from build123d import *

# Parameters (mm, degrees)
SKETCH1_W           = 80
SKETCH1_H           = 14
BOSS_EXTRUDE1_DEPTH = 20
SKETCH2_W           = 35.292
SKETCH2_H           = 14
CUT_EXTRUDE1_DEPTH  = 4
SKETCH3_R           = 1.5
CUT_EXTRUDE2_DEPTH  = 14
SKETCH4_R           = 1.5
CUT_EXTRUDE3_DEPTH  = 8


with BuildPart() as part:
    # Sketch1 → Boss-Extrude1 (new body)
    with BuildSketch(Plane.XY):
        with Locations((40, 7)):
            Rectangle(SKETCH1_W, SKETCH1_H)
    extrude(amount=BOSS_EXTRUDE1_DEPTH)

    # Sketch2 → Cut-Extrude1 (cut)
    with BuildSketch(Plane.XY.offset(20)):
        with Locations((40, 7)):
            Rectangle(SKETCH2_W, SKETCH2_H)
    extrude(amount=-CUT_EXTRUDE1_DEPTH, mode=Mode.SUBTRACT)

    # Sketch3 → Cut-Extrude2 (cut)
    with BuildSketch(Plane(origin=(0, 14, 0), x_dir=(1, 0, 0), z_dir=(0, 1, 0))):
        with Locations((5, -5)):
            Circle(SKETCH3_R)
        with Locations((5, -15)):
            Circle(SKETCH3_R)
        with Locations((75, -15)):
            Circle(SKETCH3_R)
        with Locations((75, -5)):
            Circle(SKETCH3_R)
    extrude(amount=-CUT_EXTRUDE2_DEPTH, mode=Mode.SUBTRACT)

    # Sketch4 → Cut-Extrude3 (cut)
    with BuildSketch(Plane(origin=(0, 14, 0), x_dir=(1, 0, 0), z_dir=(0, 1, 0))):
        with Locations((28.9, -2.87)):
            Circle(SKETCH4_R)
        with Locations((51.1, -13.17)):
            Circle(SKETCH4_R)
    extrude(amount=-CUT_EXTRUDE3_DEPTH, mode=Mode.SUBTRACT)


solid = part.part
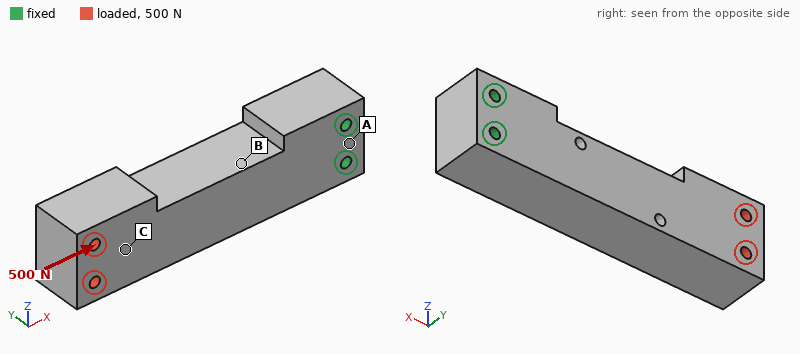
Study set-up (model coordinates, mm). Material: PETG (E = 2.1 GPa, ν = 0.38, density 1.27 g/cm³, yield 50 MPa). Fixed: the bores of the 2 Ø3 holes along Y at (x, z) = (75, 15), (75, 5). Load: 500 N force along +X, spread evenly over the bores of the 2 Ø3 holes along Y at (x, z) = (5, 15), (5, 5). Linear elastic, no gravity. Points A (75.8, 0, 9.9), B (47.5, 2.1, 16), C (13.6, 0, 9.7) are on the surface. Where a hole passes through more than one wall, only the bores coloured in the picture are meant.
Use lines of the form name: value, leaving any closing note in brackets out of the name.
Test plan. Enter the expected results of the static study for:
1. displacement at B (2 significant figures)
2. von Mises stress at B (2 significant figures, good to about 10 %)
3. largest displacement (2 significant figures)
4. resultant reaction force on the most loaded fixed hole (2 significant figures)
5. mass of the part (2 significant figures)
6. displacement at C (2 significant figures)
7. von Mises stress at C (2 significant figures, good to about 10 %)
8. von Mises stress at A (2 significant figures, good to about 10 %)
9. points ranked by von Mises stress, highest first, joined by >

displacement at B: 0.041 mm
von Mises stress at B: 4.2 MPa
largest displacement: 0.22 mm
resultant reaction force on the most loaded fixed hole: 250 N
mass of the part: 25 g
displacement at C: 0.14 mm
von Mises stress at C: 2.2 MPa
von Mises stress at A: 0.73 MPa
points ranked by von Mises stress, highest first, joined by >: B > C > A
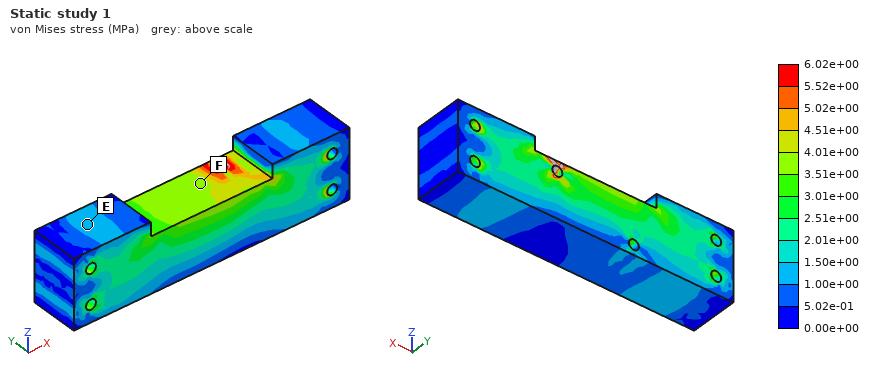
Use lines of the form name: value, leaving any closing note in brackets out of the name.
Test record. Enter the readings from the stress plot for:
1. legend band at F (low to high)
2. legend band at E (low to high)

legend band at F: 3.51e+00 to 4.01e+00 MPa
legend band at E: 1.00e+00 to 1.50e+00 MPa
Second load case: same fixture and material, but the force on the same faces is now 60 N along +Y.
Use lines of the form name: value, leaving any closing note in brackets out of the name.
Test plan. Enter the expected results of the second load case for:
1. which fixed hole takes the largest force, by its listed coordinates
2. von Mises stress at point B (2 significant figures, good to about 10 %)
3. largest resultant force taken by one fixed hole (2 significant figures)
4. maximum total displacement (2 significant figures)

which fixed hole takes the largest force, by its listed coordinates: (75, 15)
von Mises stress at point B: 3.4 MPa
largest resultant force taken by one fixed hole: 34 N
maximum total displacement: 0.97 mm
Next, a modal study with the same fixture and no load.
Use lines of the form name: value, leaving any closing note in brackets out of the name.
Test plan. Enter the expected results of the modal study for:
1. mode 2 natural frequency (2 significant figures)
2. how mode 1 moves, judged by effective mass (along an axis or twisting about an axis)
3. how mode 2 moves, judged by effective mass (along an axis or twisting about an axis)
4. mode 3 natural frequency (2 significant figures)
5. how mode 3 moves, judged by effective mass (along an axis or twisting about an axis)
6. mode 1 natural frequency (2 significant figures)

mode 2 natural frequency: 590 Hz
how mode 1 moves, judged by effective mass: along Y
how mode 2 moves, judged by effective mass: along Z
mode 3 natural frequency: 2200 Hz
how mode 3 moves, judged by effective mass: twisting about X
mode 1 natural frequency: 490 Hz
